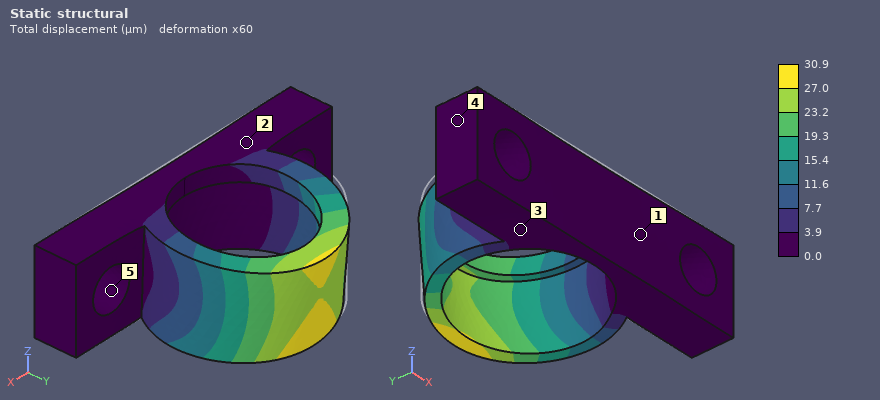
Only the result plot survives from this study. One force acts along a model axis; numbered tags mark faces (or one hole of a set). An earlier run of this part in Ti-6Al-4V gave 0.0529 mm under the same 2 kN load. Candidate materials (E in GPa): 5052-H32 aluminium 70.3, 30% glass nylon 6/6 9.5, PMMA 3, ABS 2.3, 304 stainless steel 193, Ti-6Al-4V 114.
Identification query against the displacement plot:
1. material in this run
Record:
304 stainless steel
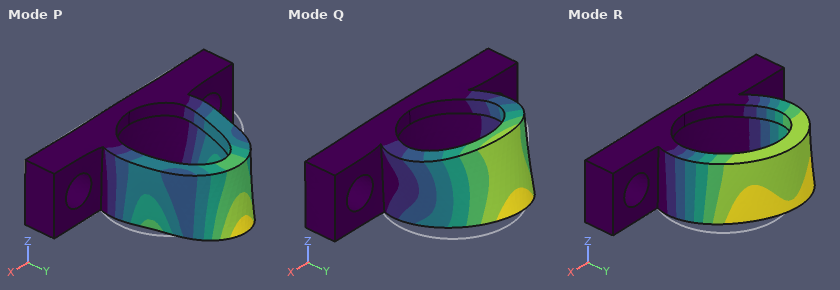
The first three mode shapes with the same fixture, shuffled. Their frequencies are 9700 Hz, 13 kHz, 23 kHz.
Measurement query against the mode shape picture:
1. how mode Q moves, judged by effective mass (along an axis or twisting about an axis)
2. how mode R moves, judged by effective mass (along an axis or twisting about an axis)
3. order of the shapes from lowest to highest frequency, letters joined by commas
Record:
along Z
along X
R, Q, P
